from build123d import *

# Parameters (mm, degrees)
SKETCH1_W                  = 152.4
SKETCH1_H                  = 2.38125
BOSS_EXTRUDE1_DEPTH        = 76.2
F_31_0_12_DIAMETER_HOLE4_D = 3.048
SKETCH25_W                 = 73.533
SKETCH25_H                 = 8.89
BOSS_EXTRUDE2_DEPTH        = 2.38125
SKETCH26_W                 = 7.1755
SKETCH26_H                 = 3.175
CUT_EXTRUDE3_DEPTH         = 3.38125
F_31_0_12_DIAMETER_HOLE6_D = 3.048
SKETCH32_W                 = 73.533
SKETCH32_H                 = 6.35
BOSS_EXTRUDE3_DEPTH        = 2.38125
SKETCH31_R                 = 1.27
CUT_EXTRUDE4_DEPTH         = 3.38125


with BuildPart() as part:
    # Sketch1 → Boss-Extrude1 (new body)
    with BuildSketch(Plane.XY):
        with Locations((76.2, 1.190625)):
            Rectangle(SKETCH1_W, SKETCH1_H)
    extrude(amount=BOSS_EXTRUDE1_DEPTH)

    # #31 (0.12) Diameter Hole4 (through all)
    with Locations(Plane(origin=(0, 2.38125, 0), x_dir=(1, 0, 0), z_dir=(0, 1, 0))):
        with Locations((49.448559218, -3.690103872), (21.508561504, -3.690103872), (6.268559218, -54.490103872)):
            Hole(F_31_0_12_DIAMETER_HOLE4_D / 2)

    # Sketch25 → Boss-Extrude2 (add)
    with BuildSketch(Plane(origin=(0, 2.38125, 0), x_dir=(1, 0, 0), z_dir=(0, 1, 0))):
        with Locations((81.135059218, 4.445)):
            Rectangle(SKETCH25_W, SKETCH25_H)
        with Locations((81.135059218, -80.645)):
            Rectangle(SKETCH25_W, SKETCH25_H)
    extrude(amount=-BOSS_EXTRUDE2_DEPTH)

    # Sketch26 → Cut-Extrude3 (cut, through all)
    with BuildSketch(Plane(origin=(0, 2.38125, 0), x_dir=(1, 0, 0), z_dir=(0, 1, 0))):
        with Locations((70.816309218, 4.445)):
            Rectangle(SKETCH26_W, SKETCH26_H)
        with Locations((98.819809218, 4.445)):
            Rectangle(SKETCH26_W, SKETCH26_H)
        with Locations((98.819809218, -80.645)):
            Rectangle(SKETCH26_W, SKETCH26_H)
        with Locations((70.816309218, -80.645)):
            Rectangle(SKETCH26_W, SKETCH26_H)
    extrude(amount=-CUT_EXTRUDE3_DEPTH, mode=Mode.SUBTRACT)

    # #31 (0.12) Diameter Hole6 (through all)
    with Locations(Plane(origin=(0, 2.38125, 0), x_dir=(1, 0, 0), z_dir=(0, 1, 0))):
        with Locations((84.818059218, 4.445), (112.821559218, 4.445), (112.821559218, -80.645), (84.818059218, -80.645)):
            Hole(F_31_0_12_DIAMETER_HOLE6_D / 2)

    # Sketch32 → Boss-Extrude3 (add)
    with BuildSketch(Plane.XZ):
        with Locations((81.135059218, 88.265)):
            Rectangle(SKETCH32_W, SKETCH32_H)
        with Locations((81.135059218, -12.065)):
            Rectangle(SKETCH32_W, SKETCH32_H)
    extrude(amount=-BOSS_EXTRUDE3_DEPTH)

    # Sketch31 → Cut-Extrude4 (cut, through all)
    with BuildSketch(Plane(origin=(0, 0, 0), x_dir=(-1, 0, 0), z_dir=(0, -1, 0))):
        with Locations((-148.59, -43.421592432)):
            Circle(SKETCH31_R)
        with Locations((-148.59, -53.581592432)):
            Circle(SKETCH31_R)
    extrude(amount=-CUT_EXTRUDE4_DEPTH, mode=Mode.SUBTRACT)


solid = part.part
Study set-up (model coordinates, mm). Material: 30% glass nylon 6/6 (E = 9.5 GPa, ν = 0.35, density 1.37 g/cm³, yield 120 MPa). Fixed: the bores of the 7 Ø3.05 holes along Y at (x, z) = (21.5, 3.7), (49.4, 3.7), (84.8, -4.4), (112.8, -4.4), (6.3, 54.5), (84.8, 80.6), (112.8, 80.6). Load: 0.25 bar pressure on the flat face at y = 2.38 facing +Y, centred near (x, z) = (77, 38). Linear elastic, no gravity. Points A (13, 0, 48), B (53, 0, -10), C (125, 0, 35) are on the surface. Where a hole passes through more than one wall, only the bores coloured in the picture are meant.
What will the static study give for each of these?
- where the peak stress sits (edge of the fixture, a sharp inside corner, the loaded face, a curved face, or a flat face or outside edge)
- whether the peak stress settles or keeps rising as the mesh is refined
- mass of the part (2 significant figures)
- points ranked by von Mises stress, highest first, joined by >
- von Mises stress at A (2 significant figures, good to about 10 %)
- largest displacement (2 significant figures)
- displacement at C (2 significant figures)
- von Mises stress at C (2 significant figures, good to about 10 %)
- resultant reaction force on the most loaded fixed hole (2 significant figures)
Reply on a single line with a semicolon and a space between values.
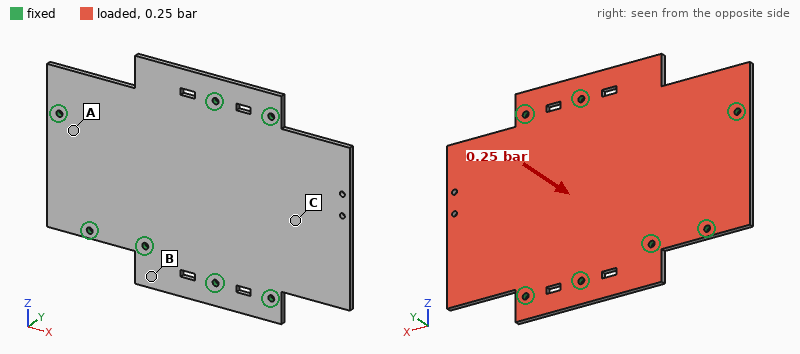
edge of the fixture; keeps rising; 45 g; C > A > B; 8.8 MPa; 2.1 mm; 0.97 mm; 14 MPa; 73 N
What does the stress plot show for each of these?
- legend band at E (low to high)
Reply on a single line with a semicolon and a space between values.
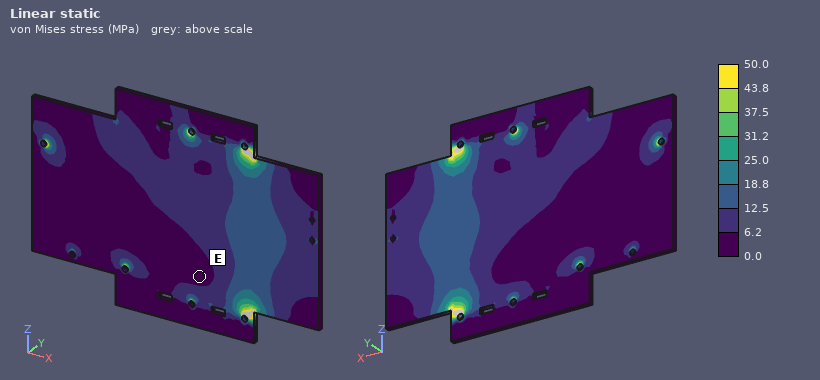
0.0 to 6.2 MPa
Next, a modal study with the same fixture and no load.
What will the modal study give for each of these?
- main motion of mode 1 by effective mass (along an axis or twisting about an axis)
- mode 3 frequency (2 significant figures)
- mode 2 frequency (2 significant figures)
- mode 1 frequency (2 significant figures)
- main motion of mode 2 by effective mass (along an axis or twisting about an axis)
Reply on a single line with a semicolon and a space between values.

along Y; 910 Hz; 840 Hz; 400 Hz; along Y
